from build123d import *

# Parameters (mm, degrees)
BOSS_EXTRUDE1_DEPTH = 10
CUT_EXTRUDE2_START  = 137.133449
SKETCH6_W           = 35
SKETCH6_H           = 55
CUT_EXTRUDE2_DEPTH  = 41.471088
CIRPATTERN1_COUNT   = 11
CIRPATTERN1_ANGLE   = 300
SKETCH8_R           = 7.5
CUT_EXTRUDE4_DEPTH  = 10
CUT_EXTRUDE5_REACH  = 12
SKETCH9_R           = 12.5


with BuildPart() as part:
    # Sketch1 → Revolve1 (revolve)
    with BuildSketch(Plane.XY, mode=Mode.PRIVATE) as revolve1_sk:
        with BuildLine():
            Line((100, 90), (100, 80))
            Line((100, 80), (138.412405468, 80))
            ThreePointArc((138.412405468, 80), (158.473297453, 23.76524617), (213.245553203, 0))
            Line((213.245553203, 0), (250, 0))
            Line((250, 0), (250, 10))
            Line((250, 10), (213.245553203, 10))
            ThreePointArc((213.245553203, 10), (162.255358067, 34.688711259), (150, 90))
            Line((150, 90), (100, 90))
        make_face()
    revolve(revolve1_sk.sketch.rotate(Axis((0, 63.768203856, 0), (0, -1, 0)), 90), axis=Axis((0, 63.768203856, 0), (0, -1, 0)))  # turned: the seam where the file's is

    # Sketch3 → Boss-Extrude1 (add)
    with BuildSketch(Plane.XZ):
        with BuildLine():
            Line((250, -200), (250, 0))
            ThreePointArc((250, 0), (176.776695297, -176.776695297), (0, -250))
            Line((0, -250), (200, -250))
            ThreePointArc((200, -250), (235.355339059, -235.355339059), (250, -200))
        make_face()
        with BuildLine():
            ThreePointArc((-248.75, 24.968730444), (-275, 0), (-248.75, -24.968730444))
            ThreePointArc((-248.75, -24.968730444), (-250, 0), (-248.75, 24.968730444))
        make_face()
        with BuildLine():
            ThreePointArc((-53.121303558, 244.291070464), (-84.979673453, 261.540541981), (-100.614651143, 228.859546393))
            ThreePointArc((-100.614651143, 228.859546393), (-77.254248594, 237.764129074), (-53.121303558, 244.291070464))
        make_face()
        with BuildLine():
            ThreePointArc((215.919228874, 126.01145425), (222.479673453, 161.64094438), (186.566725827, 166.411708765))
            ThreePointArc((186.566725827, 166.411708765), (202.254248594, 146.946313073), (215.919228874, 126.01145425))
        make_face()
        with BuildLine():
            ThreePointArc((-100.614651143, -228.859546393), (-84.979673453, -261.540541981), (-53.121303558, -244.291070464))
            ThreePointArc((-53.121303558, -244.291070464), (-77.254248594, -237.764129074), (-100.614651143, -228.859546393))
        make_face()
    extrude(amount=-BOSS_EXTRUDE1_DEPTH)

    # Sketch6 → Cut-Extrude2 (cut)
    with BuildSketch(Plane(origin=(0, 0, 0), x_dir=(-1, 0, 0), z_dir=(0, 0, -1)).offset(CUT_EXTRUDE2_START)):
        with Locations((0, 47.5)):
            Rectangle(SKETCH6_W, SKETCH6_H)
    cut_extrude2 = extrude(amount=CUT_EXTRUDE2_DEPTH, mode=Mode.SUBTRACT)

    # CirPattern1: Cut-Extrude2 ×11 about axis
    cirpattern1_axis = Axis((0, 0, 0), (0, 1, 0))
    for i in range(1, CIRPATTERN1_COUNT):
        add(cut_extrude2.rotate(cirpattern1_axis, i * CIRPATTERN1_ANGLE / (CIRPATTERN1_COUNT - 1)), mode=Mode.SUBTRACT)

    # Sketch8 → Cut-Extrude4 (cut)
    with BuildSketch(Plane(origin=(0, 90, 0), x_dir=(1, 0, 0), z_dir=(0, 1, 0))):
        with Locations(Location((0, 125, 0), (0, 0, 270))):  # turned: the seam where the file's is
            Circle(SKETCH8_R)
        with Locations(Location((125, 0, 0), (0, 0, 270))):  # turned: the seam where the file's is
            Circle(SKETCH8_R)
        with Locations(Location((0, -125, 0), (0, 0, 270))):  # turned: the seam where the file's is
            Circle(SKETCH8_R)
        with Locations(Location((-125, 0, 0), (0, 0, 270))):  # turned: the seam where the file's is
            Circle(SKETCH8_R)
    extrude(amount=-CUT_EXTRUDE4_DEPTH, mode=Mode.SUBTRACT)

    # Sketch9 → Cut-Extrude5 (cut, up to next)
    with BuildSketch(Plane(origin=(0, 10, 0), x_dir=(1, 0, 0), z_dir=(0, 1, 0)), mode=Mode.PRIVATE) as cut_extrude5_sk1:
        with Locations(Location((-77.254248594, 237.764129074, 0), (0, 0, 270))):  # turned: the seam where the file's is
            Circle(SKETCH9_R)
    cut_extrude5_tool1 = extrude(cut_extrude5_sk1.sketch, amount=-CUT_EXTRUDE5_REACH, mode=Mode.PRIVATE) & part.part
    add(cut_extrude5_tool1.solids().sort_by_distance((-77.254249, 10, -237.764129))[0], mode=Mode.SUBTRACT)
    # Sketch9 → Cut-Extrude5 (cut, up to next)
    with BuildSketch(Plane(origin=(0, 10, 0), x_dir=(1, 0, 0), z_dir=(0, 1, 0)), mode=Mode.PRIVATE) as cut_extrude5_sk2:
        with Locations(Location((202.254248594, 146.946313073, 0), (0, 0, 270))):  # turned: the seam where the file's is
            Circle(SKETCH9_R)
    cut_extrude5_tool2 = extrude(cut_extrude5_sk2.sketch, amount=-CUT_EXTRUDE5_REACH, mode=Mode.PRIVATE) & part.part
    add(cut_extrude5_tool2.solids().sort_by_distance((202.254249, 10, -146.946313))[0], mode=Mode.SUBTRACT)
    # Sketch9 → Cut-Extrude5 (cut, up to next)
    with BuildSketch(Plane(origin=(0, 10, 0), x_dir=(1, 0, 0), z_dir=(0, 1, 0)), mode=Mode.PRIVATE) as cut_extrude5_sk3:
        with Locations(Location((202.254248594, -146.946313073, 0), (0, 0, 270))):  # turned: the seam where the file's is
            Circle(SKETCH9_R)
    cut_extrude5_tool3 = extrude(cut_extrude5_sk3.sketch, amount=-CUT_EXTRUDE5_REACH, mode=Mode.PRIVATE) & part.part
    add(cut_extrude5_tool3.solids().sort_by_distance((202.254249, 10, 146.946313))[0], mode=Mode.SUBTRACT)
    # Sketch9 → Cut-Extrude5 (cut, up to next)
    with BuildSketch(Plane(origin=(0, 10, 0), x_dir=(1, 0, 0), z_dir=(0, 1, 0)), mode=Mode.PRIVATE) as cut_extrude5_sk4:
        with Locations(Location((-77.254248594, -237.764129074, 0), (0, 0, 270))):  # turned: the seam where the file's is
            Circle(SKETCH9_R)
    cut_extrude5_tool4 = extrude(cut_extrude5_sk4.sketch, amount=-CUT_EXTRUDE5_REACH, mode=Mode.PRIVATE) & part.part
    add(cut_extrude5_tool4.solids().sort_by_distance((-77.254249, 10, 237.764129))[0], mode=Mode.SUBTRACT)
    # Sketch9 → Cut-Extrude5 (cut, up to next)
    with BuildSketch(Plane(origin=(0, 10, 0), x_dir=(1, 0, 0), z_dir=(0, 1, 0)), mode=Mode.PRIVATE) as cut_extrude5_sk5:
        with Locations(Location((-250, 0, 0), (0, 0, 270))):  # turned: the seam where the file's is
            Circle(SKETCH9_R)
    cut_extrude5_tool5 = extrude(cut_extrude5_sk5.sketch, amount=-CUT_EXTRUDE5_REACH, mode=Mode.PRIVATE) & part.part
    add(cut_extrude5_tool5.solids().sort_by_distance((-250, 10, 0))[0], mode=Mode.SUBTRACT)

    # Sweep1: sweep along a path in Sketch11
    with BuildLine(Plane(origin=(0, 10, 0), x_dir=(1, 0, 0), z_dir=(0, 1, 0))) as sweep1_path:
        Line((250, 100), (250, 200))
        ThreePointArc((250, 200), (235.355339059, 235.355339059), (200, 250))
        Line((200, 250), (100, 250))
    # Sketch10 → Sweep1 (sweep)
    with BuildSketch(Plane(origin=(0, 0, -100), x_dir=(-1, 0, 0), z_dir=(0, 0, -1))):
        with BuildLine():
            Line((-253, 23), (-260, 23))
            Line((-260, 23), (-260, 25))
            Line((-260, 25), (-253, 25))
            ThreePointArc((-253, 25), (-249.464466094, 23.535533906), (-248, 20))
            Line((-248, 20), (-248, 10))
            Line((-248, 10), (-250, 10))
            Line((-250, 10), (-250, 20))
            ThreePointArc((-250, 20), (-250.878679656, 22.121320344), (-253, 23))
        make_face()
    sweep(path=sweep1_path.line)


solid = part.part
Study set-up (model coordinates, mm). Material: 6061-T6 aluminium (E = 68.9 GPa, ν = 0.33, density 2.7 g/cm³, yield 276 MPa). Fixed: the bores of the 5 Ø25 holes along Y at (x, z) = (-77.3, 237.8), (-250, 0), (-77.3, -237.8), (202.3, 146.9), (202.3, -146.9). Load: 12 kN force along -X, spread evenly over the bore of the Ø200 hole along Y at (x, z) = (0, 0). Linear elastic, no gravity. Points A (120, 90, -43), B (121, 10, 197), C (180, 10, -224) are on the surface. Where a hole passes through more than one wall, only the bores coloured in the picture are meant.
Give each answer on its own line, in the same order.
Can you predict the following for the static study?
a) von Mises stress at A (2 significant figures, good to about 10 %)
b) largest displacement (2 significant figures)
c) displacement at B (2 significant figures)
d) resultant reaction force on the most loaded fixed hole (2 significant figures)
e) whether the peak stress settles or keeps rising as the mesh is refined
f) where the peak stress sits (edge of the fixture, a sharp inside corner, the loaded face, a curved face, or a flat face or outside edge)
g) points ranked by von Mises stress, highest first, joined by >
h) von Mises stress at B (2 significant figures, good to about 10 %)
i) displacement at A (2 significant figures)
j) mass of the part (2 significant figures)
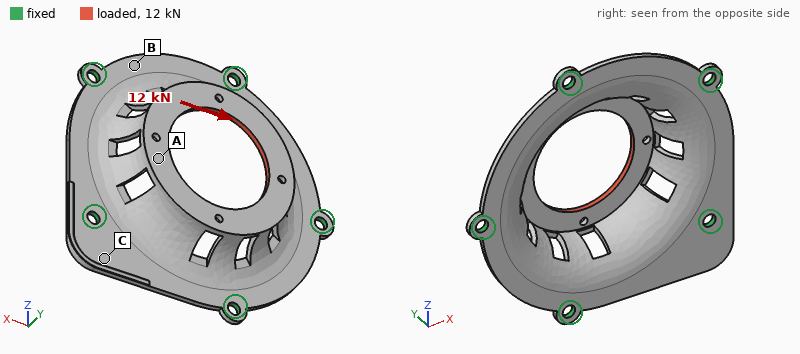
8.0 MPa
0.13 mm
0.027 mm
3.8 kN
keeps rising
edge of the fixture
A > B > C
4.2 MPa
0.096 mm
5.5 kg
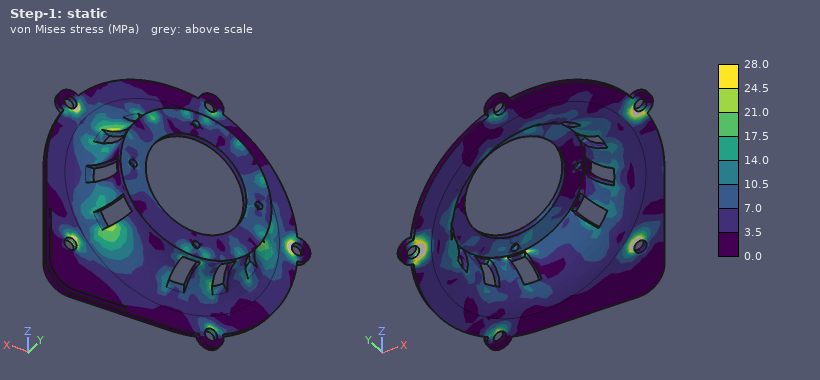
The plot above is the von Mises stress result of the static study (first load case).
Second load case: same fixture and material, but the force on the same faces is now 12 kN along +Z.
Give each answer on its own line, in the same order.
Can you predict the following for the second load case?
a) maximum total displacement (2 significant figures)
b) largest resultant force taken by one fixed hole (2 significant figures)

0.13 mm
3.8 kN
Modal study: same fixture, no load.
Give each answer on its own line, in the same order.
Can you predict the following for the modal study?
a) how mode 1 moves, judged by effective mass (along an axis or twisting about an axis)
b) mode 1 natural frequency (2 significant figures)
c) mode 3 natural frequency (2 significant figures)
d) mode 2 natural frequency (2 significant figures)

along Y
680 Hz
780 Hz
750 Hz
